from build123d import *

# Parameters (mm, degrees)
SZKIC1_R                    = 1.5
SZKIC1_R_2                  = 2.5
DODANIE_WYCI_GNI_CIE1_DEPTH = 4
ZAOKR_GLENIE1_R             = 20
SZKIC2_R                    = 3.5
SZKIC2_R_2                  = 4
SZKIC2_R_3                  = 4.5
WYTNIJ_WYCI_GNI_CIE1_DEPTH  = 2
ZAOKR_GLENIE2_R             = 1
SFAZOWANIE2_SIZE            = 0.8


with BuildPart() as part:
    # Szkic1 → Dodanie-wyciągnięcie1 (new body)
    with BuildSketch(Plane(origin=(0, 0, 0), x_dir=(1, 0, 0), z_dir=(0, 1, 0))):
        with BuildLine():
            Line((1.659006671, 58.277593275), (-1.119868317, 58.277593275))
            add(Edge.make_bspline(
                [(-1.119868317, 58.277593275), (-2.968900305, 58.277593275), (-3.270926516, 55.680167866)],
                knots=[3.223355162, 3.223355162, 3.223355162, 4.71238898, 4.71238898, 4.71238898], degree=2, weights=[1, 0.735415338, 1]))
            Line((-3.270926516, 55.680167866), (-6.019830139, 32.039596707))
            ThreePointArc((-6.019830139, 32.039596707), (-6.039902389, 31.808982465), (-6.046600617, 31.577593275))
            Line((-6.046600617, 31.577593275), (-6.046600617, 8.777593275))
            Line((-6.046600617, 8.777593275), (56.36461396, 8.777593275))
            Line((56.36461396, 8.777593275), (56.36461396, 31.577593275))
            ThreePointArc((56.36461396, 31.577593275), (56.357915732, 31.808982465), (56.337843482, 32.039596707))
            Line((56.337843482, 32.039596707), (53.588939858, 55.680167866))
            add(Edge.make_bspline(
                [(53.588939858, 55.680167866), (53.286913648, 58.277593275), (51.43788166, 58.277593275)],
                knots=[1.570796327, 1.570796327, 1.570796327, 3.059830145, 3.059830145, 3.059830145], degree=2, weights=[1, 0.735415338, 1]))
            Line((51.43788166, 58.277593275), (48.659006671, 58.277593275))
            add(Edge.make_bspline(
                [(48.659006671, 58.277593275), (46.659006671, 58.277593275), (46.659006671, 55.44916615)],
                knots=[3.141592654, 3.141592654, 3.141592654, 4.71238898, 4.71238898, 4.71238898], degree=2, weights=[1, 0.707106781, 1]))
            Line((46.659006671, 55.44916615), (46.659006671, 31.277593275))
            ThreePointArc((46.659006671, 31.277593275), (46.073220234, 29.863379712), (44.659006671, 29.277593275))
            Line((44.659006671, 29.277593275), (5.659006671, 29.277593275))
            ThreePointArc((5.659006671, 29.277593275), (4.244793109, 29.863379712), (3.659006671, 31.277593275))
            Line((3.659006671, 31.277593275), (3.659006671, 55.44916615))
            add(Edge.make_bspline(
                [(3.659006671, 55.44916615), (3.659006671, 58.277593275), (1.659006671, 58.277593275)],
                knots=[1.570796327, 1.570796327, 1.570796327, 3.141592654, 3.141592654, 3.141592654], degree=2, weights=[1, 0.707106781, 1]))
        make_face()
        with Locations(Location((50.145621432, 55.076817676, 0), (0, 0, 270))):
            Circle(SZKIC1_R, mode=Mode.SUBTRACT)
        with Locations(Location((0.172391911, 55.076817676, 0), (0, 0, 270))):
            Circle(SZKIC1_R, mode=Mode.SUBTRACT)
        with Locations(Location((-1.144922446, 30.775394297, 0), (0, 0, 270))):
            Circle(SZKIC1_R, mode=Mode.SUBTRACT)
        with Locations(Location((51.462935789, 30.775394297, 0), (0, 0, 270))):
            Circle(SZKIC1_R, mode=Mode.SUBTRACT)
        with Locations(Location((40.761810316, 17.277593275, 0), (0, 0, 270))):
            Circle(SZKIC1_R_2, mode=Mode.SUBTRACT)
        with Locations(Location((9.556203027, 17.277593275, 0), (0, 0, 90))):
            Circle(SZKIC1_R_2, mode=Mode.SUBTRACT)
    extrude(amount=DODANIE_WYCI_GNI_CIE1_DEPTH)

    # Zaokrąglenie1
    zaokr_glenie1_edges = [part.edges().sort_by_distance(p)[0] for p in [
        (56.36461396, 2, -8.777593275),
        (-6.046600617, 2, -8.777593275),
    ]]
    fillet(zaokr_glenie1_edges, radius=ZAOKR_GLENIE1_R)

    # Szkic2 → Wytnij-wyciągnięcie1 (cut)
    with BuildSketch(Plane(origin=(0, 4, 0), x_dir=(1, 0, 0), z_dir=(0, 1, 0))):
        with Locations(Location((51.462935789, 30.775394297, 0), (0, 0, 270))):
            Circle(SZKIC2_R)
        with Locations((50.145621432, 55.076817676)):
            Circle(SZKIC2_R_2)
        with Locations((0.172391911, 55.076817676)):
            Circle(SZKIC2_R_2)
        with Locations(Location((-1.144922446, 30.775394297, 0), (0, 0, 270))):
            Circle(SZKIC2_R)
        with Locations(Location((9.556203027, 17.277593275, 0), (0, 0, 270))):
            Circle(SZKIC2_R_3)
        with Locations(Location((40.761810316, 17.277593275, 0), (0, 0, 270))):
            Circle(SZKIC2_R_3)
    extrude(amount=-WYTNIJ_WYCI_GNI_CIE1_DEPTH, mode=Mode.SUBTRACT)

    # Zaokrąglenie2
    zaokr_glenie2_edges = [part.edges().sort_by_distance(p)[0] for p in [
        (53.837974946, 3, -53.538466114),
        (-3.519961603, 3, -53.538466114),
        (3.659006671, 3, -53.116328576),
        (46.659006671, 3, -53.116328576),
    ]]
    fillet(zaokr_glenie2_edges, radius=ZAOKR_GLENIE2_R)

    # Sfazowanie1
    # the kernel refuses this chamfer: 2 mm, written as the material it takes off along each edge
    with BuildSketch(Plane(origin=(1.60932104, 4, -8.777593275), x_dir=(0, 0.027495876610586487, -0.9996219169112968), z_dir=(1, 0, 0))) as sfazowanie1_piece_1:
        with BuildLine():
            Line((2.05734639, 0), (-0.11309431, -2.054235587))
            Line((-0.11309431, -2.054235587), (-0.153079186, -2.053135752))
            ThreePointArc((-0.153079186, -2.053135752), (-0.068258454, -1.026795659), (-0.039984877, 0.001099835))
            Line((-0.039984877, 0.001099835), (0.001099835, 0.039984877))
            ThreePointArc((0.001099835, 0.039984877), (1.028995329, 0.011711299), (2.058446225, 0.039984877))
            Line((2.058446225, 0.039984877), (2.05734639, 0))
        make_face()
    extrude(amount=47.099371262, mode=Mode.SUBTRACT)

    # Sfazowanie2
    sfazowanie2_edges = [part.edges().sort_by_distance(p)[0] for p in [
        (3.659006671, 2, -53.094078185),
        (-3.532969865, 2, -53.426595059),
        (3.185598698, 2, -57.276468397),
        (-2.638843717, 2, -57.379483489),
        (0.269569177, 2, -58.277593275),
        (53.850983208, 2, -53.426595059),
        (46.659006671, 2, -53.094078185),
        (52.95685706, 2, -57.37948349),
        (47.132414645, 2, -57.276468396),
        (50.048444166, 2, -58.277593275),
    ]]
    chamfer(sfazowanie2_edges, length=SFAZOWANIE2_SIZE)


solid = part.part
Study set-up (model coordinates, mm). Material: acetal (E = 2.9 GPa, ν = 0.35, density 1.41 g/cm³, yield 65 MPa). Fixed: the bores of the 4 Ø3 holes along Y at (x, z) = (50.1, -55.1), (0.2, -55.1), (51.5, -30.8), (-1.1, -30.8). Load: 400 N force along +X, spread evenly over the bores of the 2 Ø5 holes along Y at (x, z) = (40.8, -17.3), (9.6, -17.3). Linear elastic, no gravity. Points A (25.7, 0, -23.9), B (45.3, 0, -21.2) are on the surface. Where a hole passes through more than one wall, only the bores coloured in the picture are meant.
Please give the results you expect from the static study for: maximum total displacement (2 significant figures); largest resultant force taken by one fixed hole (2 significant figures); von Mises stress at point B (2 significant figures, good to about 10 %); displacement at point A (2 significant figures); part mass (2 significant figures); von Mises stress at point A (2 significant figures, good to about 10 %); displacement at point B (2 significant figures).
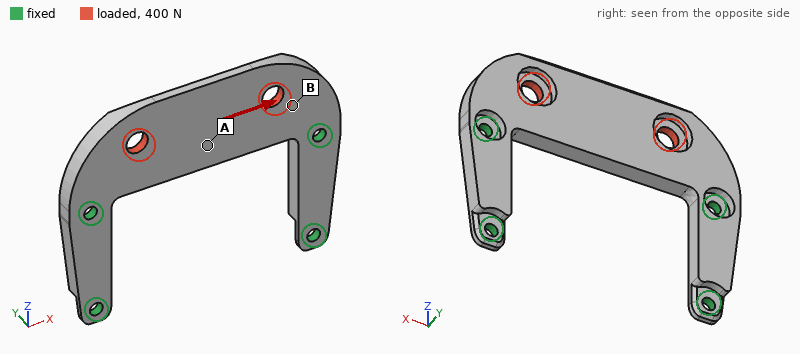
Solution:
0.12 mm
220 N
6.5 MPa
0.071 mm
7.8 g
2.8 MPa
0.078 mm
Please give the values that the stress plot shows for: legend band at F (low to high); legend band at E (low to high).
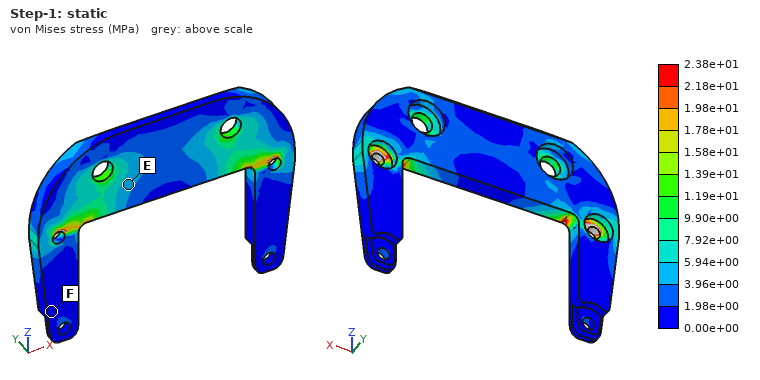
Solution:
0.00e+00 to 1.98e+00 MPa
3.96e+00 to 5.94e+00 MPa
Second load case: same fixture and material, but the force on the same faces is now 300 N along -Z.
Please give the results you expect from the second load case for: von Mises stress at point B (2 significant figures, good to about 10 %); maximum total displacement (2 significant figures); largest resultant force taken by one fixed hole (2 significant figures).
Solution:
6.9 MPa
0.16 mm
160 N
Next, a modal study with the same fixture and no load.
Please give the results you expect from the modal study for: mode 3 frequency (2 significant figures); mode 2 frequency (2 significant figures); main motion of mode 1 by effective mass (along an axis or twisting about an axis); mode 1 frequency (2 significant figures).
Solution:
2300 Hz
2300 Hz
along Y
850 Hz
